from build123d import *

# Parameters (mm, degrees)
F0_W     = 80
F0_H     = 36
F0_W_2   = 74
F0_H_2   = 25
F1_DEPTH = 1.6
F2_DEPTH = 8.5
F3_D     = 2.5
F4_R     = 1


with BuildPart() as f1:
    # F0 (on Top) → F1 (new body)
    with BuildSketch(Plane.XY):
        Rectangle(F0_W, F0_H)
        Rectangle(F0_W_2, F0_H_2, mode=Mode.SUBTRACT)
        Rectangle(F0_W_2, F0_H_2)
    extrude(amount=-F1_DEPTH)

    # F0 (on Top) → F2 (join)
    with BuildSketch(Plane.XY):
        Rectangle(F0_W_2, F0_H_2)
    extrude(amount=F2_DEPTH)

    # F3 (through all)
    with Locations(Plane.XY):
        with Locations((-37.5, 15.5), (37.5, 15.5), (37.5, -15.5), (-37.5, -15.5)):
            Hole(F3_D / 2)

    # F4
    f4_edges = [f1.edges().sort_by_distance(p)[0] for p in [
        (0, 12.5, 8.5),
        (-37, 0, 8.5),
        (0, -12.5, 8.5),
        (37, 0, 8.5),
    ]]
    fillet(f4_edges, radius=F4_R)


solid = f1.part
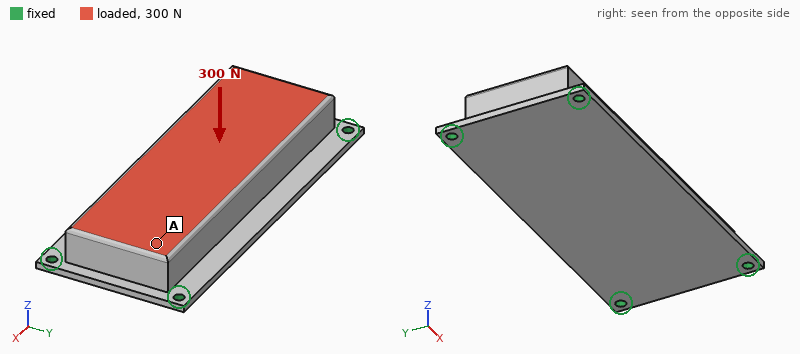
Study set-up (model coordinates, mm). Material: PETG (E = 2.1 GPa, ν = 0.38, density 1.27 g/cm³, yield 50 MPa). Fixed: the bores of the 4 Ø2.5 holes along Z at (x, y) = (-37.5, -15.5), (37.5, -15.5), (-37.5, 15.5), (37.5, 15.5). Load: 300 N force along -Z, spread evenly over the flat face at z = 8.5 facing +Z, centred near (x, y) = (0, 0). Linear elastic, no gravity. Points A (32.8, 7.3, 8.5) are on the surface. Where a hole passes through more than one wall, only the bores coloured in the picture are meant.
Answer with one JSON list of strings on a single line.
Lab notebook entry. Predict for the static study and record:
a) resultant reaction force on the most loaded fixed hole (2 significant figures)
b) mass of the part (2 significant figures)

["120 N", "26 g"]
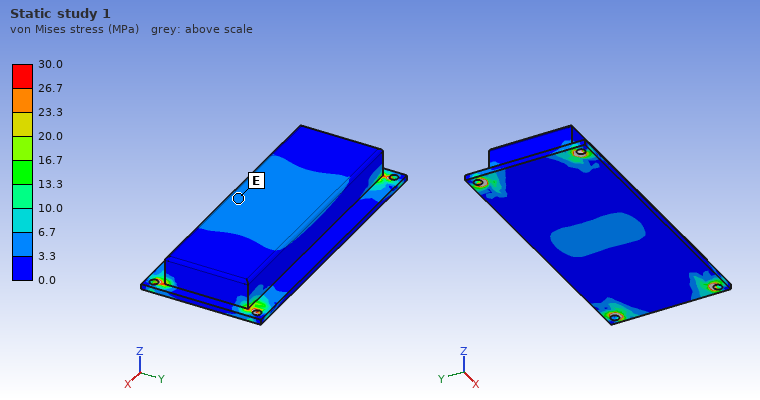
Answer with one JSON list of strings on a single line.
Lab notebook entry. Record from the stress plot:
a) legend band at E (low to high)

["3.3 to 6.7 MPa"]
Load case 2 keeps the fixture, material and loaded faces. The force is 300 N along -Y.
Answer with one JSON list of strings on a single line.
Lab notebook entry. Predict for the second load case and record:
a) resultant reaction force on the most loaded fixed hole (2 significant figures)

["110 N"]
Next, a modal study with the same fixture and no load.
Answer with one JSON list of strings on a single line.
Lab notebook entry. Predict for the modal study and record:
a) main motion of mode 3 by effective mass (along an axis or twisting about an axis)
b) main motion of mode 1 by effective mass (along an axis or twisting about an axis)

["twisting about Y", "along Z"]
